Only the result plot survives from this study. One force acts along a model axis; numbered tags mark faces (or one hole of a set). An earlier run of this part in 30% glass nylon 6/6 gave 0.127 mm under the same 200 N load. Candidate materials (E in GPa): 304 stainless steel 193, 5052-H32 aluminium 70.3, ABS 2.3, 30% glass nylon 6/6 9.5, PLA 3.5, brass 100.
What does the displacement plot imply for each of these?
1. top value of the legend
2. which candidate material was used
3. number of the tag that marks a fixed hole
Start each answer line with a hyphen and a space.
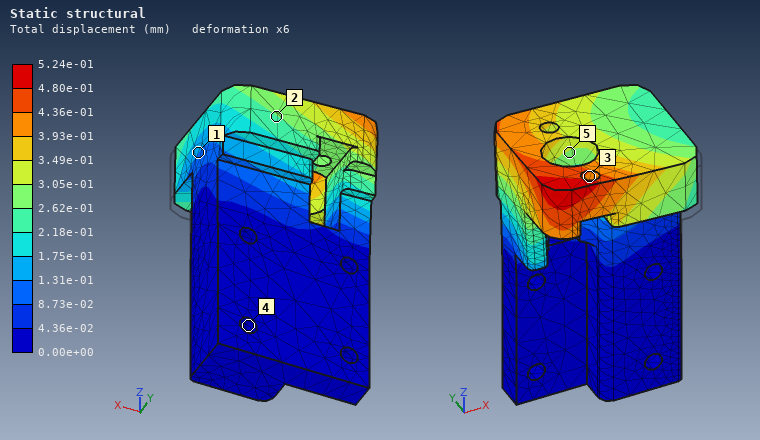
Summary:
- 5.24e-01 mm
- ABS
- 4
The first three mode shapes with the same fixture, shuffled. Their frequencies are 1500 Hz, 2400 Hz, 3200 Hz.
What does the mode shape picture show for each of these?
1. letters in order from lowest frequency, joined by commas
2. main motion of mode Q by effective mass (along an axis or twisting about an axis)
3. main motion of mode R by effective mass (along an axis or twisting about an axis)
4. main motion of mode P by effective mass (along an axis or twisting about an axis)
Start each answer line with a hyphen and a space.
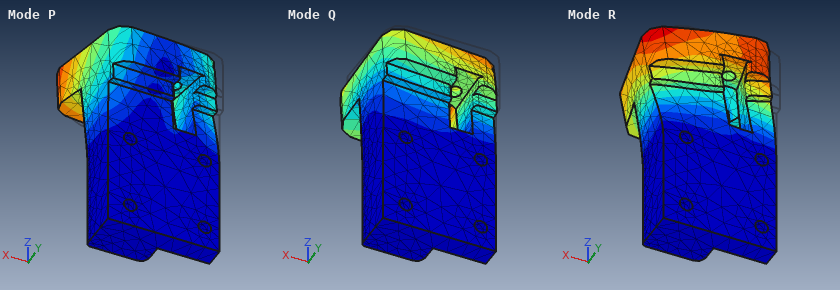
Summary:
- Q, P, R
- along Y
- along X
- along X
